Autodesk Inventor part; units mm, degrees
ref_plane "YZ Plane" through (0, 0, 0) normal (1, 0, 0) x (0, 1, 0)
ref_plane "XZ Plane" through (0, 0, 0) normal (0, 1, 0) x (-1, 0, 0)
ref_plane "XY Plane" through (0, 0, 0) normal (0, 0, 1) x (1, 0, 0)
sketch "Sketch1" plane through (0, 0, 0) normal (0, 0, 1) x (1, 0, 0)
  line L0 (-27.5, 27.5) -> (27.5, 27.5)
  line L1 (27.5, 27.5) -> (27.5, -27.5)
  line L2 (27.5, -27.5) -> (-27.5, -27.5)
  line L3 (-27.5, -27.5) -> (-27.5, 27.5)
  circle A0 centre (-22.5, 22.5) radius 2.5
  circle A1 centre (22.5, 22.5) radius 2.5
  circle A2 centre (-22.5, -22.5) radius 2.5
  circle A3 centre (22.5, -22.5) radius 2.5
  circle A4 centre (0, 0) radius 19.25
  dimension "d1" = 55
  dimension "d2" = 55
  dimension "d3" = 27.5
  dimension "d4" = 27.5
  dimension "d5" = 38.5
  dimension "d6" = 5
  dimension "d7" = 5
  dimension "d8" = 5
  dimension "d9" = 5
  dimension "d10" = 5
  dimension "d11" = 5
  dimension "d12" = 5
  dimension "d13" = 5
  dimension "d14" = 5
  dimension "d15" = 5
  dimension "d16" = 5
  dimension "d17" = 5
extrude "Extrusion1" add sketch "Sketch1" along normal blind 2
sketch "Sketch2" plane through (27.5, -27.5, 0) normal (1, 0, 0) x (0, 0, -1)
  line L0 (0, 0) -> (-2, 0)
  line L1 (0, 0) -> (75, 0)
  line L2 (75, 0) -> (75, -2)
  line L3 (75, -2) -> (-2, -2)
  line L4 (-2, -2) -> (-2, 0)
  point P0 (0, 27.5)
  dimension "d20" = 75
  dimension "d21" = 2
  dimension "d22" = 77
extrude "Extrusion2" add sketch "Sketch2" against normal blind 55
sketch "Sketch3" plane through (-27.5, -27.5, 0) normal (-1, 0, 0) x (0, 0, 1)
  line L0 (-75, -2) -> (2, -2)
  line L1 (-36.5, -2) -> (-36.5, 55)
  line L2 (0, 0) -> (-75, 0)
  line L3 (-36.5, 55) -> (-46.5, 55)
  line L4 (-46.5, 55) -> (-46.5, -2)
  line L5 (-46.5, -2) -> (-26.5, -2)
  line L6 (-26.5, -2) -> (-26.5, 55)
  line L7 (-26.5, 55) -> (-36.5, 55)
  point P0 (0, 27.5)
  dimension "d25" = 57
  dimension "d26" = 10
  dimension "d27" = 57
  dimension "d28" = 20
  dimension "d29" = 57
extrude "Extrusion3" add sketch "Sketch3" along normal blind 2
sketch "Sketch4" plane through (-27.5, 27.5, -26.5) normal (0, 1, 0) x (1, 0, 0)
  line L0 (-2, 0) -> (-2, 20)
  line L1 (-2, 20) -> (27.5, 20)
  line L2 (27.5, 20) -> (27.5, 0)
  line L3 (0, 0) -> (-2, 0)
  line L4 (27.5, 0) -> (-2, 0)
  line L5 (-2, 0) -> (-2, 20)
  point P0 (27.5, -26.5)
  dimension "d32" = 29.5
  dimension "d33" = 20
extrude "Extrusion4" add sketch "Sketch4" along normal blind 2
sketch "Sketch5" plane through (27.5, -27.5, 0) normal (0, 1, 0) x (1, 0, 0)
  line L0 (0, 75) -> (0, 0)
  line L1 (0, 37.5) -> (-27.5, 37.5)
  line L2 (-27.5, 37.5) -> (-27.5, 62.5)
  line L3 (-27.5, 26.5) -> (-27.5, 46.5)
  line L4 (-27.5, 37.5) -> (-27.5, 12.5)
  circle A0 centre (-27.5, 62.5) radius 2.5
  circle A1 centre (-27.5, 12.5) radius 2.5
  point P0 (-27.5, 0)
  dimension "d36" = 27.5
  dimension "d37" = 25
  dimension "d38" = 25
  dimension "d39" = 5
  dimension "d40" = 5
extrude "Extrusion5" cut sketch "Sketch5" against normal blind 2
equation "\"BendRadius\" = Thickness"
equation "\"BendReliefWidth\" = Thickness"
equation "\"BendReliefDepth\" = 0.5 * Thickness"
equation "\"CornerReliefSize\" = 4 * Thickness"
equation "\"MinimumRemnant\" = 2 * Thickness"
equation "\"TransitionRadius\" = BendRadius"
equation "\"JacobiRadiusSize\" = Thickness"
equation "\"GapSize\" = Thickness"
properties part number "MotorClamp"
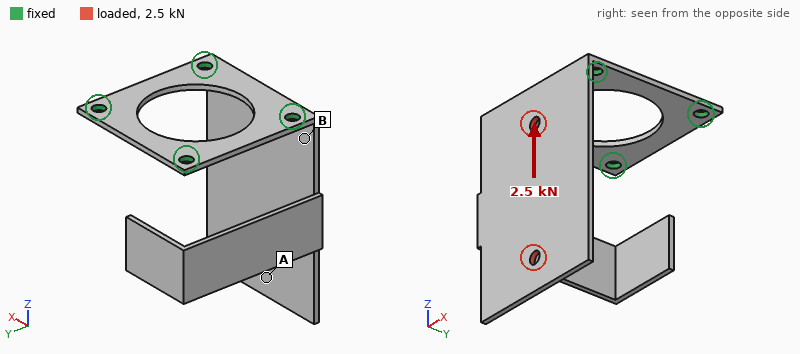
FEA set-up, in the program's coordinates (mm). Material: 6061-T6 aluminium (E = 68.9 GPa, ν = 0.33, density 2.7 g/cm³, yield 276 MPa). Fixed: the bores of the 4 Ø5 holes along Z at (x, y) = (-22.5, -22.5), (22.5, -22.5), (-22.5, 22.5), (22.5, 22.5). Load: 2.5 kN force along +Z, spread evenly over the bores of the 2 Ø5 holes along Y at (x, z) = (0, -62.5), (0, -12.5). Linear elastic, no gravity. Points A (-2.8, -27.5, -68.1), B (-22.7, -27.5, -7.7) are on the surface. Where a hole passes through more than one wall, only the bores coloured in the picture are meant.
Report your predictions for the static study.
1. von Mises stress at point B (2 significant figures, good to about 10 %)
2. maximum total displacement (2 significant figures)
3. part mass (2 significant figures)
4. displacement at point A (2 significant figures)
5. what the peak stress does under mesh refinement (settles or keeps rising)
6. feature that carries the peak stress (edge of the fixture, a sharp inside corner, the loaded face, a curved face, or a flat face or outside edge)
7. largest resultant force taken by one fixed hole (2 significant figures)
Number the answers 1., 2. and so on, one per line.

1. 56 MPa
2. 1.1 mm
3. 42 g
4. 1.0 mm
5. keeps rising
6. edge of the fixture
7. 1.3 kN
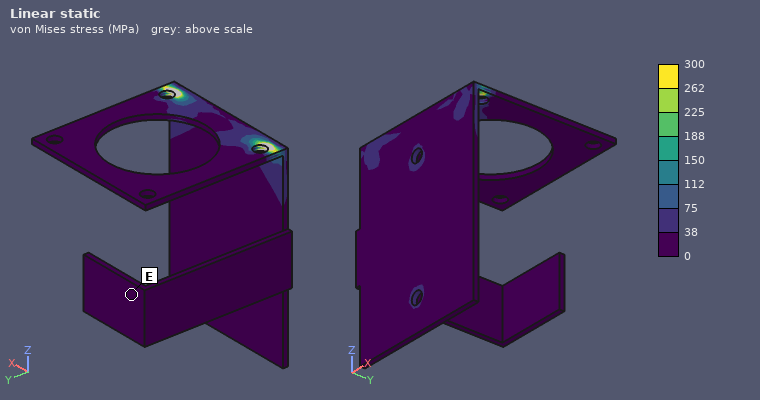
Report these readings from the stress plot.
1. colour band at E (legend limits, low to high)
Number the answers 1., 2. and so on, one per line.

1. 0 to 38 MPa
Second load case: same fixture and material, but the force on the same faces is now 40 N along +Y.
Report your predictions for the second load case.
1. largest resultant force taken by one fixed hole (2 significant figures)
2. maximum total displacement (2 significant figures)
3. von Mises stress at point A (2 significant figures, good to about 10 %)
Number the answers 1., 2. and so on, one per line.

1. 19 N
2. 1.2 mm
3. 8.2 MPa
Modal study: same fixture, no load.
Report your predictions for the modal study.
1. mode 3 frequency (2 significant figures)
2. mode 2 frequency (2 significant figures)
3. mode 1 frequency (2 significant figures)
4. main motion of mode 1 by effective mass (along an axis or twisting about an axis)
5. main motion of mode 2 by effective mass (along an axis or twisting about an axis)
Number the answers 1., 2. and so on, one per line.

1. 520 Hz
2. 210 Hz
3. 180 Hz
4. along Y
5. along X
